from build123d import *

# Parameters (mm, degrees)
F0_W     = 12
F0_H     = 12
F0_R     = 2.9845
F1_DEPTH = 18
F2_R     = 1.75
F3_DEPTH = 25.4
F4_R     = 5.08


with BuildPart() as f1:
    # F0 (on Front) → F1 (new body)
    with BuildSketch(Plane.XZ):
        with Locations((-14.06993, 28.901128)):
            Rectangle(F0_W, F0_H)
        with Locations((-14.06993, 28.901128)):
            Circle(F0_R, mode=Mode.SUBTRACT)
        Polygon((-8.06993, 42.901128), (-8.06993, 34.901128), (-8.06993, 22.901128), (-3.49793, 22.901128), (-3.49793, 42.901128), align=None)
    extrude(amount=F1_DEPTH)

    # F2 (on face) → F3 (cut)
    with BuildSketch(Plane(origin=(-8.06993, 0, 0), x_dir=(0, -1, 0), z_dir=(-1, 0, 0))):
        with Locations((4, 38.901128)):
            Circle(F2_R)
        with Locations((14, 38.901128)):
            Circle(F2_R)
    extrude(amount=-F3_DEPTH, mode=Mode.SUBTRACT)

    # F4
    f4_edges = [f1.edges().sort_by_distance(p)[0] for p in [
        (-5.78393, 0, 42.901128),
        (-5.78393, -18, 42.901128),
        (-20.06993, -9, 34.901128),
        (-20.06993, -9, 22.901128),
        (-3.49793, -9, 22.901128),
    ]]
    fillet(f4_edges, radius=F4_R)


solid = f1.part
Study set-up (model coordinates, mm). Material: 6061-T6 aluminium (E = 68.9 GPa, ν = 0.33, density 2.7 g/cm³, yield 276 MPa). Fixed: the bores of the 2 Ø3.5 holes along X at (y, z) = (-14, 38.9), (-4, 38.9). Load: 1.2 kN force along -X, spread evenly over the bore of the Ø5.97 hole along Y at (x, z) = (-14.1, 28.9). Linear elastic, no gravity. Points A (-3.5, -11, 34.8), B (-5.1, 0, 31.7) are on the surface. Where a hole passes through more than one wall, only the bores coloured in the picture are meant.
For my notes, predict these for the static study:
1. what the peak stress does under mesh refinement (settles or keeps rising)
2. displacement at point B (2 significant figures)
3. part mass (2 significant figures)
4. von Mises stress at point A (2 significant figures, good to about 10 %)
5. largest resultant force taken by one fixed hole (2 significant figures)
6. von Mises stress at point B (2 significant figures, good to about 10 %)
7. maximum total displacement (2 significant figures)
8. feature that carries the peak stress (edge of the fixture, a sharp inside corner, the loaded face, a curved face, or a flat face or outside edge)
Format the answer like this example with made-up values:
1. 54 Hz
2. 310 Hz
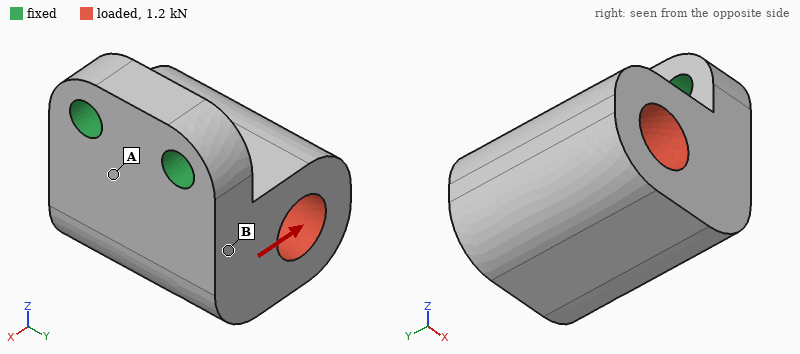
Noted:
1. keeps rising
2. 20 µm
3. 8.9 g
4. 84 MPa
5. 600 N
6. 34 MPa
7. 80 µm
8. edge of the fixture
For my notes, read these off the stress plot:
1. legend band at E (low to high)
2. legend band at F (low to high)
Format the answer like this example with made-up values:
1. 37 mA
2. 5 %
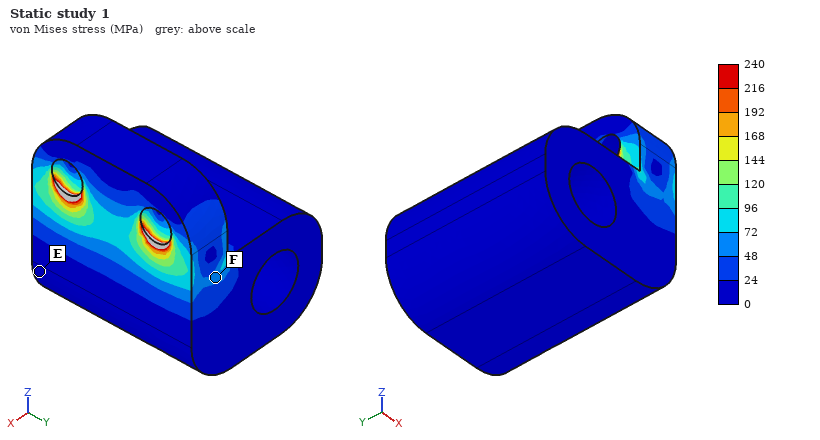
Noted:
1. 0 to 24 MPa
2. 48 to 72 MPa
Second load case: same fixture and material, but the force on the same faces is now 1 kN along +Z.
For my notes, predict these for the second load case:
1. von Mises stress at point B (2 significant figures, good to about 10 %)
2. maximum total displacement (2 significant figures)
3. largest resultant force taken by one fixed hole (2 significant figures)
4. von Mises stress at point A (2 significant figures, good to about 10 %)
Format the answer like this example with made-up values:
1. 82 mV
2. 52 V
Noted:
1. 36 MPa
2. 81 µm
3. 510 N
4. 88 MPa
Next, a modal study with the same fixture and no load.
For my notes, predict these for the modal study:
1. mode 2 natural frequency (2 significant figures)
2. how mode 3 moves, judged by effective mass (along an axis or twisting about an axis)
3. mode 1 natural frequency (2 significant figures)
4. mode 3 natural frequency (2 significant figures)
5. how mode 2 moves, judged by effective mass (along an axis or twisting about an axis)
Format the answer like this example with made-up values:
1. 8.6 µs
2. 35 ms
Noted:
1. 16 kHz
2. along Y
3. 7500 Hz
4. 26 kHz
5. along Y
